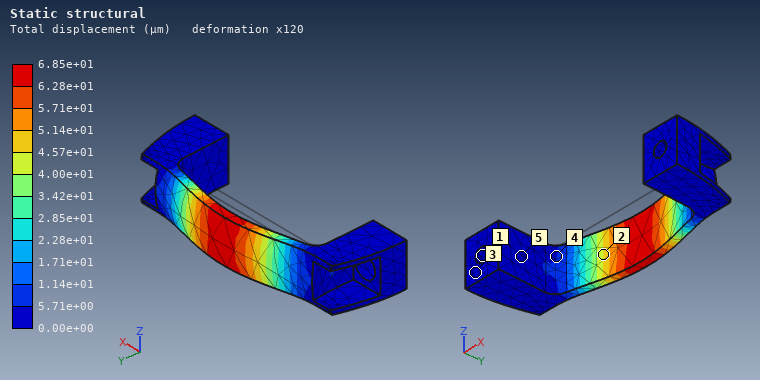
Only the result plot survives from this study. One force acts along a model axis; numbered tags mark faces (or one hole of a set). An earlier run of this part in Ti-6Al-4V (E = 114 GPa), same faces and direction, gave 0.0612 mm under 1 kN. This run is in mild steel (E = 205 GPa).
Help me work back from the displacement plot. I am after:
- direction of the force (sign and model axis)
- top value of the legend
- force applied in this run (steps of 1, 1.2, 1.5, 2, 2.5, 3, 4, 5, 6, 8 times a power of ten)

+Y
6.85e+01 µm
2 kN
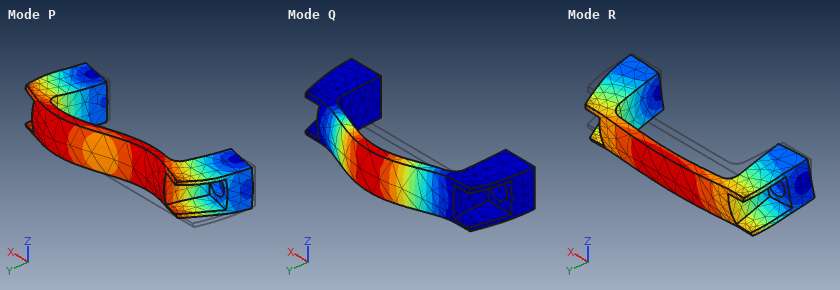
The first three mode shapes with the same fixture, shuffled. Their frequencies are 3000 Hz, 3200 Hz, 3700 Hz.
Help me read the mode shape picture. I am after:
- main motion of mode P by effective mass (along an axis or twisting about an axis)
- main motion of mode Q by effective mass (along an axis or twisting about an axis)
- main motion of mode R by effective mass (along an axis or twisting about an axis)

along X
along Y
along Z
